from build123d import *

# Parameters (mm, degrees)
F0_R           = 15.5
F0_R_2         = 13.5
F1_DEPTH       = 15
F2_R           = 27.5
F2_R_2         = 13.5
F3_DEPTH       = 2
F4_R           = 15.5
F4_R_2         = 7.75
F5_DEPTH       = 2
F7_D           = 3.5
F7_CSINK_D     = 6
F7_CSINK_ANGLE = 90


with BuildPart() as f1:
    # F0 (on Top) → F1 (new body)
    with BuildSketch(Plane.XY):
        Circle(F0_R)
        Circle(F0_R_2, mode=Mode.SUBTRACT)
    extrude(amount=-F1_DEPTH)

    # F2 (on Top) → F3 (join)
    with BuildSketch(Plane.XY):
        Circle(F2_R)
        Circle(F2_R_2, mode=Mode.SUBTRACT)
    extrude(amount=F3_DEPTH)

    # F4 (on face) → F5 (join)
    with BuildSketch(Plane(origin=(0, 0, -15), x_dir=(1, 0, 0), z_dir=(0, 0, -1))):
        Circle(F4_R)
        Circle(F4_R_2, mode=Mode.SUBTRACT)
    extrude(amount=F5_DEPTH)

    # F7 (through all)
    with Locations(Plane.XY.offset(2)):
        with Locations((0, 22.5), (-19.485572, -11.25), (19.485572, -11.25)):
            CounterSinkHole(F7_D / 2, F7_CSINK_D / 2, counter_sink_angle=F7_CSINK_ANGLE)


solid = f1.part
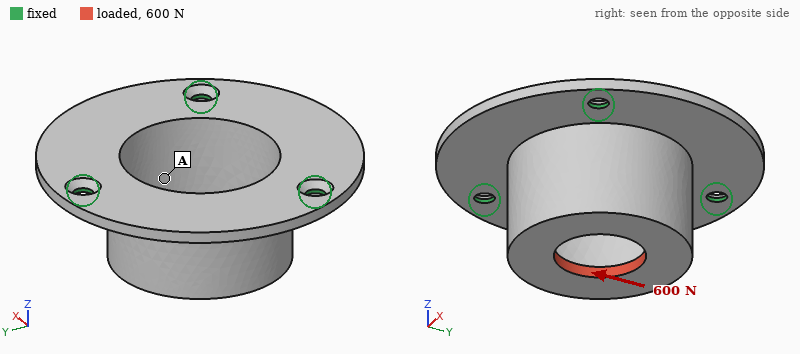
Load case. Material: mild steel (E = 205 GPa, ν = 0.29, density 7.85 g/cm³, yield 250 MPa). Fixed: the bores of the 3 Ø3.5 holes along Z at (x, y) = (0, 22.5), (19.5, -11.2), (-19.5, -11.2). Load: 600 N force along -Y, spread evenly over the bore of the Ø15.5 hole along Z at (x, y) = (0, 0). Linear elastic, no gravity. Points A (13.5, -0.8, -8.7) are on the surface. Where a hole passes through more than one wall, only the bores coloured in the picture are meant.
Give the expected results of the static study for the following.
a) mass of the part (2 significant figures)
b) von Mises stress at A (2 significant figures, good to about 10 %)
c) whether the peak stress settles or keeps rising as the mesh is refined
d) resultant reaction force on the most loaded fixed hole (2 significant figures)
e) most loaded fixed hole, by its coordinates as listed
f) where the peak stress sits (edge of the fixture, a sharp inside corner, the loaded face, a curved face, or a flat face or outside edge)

58 g
15 MPa
keeps rising
350 N
(0, 22.5)
edge of the fixture
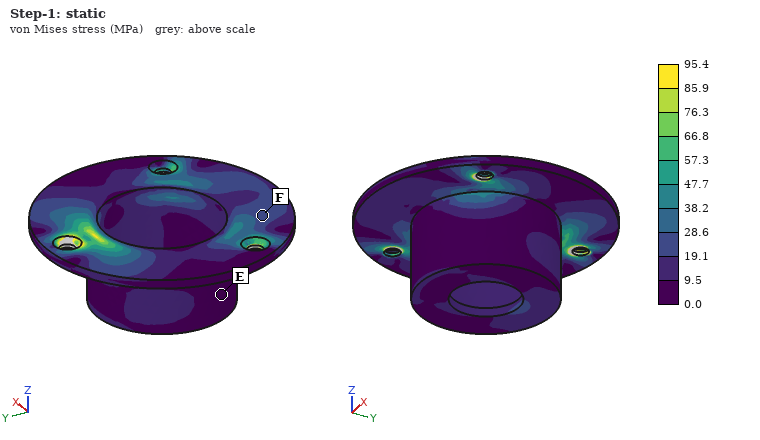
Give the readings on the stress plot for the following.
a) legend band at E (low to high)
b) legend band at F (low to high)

0.0 to 9.5 MPa
19.1 to 28.6 MPa
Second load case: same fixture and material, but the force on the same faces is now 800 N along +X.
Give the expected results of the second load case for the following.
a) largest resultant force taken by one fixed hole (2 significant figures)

440 N
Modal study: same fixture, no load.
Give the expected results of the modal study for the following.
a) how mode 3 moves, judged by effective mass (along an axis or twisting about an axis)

along Z
